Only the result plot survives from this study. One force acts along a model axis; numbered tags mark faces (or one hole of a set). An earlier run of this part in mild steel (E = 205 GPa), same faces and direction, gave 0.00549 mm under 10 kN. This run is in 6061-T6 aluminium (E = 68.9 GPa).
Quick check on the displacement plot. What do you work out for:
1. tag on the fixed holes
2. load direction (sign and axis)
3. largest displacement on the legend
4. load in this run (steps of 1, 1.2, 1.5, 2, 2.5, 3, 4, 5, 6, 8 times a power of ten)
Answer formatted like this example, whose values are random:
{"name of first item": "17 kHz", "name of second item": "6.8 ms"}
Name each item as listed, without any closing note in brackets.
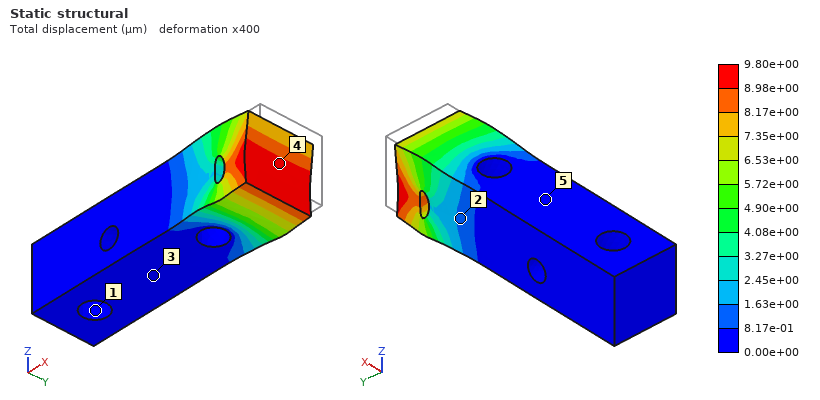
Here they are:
{"tag on the fixed holes": "1", "load direction": "-X", "largest displacement on the legend": "9.80e+00 µm", "load in this run": "6 kN"}
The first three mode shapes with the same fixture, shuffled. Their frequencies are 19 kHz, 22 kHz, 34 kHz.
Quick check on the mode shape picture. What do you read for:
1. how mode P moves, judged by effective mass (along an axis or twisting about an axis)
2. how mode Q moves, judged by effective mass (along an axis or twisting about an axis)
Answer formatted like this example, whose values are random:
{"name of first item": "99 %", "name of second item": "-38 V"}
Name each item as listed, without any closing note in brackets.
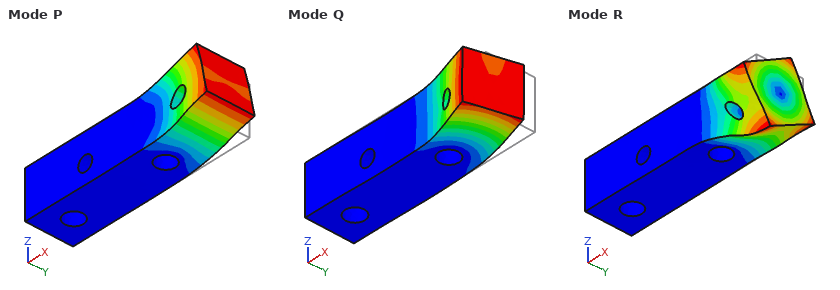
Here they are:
{"how mode P moves, judged by effective mass": "along Z", "how mode Q moves, judged by effective mass": "along Y"}
